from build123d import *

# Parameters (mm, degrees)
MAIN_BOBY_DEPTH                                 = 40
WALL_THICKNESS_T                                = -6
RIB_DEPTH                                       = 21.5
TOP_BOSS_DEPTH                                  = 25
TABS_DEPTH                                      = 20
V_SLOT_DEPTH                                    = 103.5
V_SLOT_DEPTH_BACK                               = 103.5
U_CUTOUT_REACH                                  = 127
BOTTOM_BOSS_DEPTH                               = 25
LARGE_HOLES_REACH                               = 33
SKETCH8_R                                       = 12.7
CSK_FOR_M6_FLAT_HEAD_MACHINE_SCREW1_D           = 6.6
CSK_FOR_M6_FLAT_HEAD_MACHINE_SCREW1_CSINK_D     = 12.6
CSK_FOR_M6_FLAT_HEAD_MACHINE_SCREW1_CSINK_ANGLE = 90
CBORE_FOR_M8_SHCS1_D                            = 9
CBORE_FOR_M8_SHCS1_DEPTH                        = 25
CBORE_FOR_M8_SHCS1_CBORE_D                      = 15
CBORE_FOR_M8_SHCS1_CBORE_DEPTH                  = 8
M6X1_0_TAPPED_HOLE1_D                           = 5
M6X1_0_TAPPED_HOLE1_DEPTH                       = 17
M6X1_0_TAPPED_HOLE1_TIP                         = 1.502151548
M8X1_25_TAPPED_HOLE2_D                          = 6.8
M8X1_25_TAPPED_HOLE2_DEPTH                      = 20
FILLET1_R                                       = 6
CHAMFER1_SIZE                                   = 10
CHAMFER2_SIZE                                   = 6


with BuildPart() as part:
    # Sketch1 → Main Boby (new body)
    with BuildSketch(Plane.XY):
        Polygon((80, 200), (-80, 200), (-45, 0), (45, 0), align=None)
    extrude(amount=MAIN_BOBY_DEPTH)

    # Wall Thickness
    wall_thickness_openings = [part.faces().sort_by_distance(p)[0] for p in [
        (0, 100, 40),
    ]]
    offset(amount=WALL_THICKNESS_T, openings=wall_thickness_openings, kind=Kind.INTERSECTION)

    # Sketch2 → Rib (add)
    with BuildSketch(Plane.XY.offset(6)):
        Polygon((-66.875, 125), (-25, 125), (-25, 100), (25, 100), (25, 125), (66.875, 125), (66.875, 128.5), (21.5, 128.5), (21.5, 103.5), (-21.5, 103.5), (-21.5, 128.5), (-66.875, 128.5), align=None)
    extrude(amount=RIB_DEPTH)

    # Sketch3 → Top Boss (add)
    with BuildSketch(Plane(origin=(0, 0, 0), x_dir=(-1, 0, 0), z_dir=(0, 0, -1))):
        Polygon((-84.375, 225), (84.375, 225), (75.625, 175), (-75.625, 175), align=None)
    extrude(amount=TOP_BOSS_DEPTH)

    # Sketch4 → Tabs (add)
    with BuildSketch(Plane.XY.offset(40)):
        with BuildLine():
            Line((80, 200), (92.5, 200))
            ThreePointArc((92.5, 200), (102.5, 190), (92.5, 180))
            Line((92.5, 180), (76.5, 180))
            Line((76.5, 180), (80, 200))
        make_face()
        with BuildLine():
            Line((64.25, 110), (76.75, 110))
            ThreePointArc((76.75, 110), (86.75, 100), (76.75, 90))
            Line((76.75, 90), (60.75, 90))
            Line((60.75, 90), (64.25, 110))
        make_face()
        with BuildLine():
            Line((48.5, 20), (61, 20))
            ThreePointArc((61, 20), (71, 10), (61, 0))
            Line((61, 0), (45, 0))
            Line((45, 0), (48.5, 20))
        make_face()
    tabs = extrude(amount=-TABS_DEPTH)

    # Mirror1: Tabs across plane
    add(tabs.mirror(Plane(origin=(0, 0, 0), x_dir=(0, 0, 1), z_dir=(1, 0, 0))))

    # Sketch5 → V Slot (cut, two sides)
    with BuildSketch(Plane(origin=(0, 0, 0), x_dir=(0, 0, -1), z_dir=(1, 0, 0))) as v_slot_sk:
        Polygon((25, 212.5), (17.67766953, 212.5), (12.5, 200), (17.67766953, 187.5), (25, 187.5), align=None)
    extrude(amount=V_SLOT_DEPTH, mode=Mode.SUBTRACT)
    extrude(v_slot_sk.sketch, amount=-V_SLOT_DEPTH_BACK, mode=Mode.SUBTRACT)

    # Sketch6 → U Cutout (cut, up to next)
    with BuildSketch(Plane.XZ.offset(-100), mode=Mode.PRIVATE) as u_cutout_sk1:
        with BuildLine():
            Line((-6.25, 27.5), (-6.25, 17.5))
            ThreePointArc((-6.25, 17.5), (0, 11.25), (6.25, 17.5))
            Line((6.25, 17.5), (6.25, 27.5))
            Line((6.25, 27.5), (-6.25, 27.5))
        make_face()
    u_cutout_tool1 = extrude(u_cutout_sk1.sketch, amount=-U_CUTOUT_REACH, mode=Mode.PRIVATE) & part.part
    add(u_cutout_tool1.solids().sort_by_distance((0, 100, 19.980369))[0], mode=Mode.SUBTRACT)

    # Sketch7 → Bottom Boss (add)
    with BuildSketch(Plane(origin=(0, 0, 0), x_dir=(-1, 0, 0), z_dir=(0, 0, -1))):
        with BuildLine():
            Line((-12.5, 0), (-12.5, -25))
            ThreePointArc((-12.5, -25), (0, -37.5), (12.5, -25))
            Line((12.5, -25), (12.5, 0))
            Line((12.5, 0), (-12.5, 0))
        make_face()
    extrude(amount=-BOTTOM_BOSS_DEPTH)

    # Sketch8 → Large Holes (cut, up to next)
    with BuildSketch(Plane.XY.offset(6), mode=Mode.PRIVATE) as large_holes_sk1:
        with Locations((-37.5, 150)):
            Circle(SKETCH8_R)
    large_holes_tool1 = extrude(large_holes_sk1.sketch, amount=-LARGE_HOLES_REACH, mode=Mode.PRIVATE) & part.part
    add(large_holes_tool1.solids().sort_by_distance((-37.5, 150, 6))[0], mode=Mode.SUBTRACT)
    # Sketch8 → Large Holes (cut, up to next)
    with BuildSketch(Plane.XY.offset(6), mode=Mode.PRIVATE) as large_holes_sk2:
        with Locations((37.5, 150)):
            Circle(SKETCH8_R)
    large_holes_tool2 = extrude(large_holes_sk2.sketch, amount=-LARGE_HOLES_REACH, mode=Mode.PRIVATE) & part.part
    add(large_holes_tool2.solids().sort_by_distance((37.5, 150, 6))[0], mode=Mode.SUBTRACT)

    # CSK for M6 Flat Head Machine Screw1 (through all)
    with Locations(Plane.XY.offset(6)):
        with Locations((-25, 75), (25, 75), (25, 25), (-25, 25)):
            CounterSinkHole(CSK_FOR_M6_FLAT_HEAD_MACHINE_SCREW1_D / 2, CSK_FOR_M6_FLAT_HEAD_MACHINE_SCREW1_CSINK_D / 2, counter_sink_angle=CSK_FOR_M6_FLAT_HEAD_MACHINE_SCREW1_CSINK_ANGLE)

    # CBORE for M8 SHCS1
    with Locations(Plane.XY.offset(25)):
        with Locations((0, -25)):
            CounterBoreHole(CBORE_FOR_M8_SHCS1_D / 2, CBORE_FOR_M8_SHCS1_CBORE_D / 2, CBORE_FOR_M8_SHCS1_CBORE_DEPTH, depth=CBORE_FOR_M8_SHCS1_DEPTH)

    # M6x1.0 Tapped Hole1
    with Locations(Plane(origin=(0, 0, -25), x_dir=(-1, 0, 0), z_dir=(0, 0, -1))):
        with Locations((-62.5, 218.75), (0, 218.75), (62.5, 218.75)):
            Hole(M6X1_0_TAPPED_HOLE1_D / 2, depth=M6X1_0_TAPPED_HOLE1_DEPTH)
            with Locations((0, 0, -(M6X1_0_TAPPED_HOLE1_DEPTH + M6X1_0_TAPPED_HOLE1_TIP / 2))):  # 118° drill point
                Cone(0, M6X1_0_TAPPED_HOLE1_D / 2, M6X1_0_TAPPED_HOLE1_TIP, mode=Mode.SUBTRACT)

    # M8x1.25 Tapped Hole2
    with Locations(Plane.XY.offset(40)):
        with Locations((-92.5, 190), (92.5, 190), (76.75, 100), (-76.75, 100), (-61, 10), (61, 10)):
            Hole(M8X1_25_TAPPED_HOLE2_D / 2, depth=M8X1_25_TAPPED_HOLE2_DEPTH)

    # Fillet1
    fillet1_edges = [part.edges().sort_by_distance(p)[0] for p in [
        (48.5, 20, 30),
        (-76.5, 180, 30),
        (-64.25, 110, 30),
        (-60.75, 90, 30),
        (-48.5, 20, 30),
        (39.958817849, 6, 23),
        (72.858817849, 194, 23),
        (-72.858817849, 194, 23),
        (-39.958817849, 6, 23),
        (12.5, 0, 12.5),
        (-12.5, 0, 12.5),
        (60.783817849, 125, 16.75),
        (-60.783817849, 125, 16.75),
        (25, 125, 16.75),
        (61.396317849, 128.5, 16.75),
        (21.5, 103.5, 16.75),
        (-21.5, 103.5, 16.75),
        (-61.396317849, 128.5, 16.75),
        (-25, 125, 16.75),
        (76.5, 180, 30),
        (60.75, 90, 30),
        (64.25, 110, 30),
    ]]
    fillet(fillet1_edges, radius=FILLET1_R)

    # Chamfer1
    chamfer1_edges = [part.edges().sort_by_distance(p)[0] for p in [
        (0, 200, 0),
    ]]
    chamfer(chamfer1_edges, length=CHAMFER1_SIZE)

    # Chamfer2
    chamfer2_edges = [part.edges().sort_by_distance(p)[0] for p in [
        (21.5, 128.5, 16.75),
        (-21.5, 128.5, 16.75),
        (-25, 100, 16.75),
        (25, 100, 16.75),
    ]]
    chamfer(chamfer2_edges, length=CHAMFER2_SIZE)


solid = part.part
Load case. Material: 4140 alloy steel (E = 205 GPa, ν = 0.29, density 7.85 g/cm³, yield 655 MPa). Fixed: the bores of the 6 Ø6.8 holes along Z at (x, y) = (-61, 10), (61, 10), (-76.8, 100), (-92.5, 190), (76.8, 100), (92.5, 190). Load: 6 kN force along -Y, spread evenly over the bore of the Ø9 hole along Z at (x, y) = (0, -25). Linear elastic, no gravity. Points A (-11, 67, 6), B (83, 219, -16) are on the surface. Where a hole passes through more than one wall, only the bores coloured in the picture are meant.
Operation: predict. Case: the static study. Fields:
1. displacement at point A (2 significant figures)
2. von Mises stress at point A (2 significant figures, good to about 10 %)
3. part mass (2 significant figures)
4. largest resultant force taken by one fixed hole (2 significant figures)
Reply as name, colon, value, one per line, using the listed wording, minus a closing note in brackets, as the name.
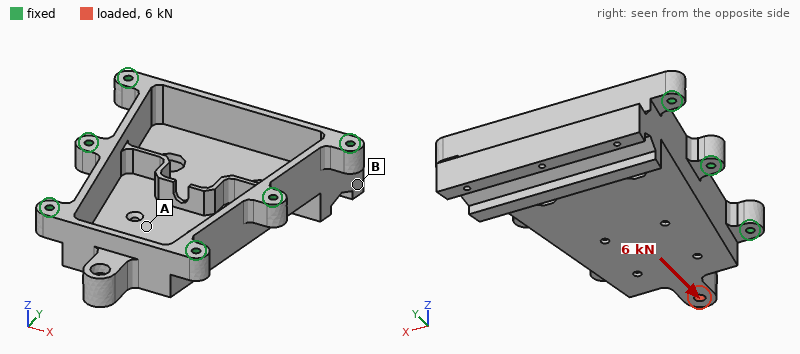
displacement at point A: 3.8 µm
von Mises stress at point A: 6.1 MPa
part mass: 4.1 kg
largest resultant force taken by one fixed hole: 1.5 kN
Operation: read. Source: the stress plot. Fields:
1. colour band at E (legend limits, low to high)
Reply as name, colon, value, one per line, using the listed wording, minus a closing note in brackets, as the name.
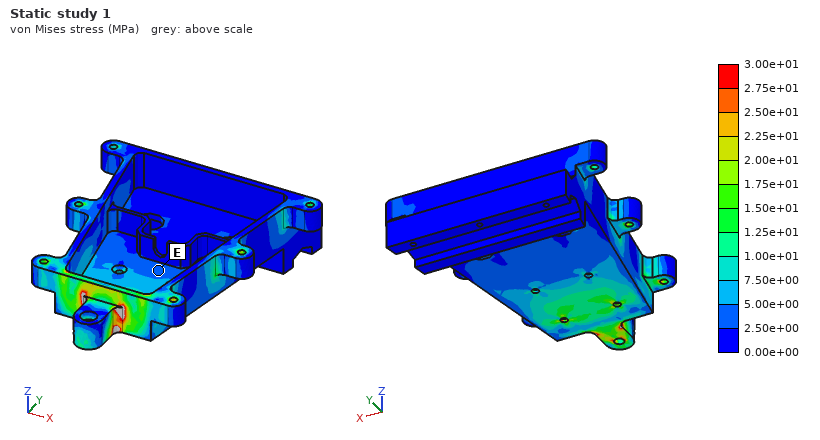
colour band at E: 2.50e+00 to 5.00e+00 MPa
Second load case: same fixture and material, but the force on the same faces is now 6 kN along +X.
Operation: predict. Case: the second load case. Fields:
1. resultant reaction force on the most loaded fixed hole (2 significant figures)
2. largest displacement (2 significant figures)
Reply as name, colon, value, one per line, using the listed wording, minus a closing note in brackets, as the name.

resultant reaction force on the most loaded fixed hole: 3.2 kN
largest displacement: 41 µm
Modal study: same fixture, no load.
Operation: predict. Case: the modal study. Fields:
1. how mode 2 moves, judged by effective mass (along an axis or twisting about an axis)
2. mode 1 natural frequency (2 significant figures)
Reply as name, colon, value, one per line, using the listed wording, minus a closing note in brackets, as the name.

how mode 2 moves, judged by effective mass: along Z
mode 1 natural frequency: 2500 Hz
